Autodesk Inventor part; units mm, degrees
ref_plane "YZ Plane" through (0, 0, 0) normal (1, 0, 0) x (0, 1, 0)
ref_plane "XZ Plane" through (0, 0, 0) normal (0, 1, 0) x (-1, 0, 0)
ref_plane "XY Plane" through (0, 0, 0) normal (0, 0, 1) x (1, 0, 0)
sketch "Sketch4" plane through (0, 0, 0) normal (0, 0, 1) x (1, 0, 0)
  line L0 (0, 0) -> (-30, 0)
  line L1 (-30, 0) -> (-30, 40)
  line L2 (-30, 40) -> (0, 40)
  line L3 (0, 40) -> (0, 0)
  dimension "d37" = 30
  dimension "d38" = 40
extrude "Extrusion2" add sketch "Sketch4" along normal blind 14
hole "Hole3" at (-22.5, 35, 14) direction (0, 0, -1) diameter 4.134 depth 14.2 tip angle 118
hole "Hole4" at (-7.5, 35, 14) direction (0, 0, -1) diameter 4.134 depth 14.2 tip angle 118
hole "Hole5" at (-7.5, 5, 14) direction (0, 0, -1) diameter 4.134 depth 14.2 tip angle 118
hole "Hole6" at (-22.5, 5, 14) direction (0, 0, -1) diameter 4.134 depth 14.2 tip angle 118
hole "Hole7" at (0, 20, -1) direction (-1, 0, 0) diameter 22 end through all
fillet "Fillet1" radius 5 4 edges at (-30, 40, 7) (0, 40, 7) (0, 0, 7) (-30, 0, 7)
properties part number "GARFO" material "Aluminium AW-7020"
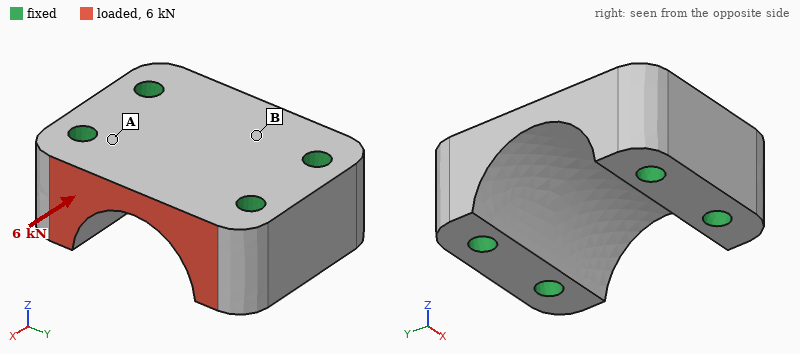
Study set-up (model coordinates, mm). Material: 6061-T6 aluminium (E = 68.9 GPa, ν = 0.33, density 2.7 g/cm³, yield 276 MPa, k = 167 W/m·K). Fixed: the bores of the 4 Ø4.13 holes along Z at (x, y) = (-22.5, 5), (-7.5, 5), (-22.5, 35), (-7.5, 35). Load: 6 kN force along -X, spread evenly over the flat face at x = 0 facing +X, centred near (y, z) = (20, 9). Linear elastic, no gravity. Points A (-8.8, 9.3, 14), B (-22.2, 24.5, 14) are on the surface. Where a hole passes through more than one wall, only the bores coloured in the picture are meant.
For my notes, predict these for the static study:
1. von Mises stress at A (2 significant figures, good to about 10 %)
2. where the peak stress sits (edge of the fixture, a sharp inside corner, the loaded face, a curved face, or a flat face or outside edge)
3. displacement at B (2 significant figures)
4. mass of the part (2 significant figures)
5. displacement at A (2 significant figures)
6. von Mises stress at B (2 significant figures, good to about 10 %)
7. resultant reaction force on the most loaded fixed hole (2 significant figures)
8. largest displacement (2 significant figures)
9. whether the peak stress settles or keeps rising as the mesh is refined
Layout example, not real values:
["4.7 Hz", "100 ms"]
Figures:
["23 MPa", "edge of the fixture", "2.1 µm", "29 g", "1.9 µm", "7.6 MPa", "2.3 kN", "8.2 µm", "keeps rising"]
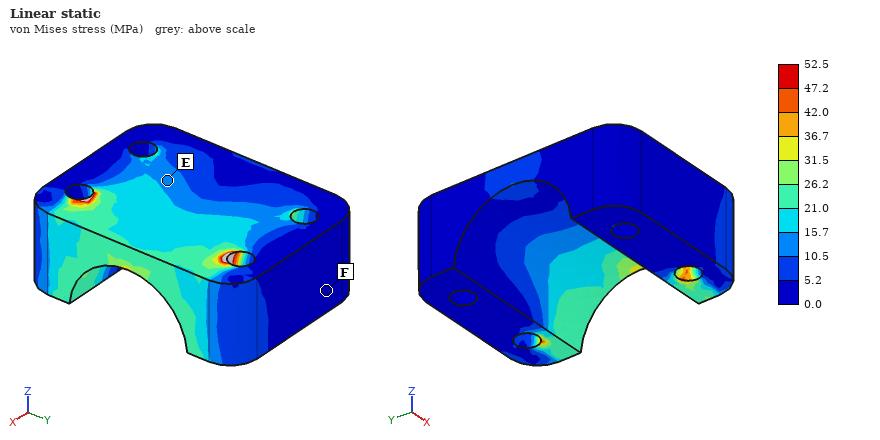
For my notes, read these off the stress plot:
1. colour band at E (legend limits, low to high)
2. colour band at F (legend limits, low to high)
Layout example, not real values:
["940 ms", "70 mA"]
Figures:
["10.5 to 15.7 MPa", "0.0 to 5.2 MPa"]
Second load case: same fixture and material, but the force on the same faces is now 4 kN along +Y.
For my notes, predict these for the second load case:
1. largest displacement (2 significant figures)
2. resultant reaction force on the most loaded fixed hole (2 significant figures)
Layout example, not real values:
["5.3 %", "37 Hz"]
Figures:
["6.3 µm", "2.1 kN"]
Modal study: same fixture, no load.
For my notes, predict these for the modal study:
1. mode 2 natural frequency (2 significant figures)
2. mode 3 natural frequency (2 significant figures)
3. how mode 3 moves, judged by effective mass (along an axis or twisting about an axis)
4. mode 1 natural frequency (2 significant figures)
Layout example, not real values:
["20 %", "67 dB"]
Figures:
["49 kHz", "59 kHz", "along X", "48 kHz"]
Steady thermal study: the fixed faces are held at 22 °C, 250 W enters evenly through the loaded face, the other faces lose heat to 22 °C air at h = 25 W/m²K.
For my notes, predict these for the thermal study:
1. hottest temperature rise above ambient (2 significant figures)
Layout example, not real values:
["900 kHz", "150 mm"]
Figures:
["60 K"]
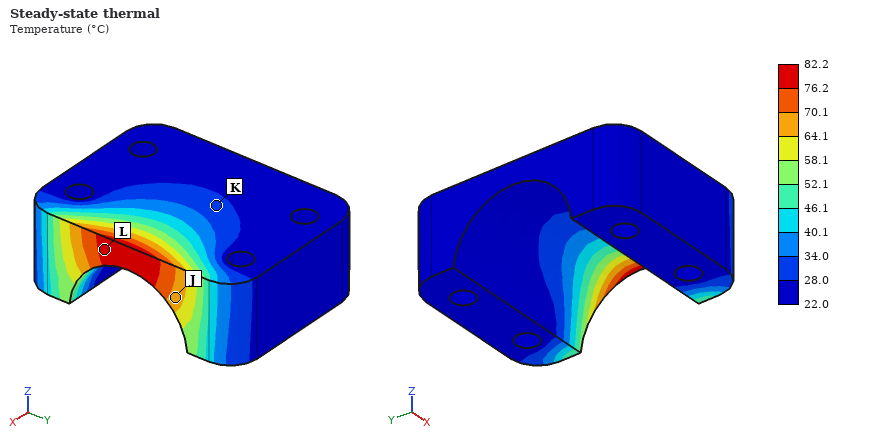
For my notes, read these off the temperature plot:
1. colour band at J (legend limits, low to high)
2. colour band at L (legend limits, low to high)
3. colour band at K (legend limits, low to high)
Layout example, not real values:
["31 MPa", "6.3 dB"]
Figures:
["64.1 to 70.1 °C", "76.2 to 82.2 °C", "28.0 to 34.0 °C"]
